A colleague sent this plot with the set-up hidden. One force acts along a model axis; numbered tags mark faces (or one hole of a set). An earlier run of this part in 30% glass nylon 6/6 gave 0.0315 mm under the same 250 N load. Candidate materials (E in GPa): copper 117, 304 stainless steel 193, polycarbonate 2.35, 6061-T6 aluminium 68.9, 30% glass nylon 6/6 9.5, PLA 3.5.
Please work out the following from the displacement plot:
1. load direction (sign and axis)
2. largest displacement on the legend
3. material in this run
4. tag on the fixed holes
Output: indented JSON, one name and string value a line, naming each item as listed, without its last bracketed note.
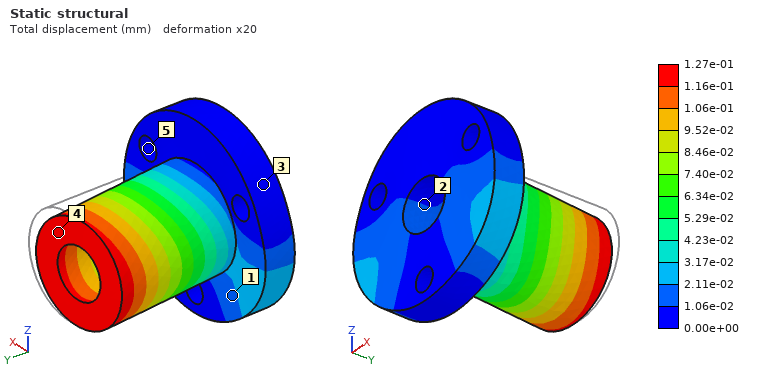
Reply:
{
  "load direction": "-X",
  "largest displacement on the legend": "1.27e-01 mm",
  "material in this run": "polycarbonate",
  "tag on the fixed holes": "5"
}
